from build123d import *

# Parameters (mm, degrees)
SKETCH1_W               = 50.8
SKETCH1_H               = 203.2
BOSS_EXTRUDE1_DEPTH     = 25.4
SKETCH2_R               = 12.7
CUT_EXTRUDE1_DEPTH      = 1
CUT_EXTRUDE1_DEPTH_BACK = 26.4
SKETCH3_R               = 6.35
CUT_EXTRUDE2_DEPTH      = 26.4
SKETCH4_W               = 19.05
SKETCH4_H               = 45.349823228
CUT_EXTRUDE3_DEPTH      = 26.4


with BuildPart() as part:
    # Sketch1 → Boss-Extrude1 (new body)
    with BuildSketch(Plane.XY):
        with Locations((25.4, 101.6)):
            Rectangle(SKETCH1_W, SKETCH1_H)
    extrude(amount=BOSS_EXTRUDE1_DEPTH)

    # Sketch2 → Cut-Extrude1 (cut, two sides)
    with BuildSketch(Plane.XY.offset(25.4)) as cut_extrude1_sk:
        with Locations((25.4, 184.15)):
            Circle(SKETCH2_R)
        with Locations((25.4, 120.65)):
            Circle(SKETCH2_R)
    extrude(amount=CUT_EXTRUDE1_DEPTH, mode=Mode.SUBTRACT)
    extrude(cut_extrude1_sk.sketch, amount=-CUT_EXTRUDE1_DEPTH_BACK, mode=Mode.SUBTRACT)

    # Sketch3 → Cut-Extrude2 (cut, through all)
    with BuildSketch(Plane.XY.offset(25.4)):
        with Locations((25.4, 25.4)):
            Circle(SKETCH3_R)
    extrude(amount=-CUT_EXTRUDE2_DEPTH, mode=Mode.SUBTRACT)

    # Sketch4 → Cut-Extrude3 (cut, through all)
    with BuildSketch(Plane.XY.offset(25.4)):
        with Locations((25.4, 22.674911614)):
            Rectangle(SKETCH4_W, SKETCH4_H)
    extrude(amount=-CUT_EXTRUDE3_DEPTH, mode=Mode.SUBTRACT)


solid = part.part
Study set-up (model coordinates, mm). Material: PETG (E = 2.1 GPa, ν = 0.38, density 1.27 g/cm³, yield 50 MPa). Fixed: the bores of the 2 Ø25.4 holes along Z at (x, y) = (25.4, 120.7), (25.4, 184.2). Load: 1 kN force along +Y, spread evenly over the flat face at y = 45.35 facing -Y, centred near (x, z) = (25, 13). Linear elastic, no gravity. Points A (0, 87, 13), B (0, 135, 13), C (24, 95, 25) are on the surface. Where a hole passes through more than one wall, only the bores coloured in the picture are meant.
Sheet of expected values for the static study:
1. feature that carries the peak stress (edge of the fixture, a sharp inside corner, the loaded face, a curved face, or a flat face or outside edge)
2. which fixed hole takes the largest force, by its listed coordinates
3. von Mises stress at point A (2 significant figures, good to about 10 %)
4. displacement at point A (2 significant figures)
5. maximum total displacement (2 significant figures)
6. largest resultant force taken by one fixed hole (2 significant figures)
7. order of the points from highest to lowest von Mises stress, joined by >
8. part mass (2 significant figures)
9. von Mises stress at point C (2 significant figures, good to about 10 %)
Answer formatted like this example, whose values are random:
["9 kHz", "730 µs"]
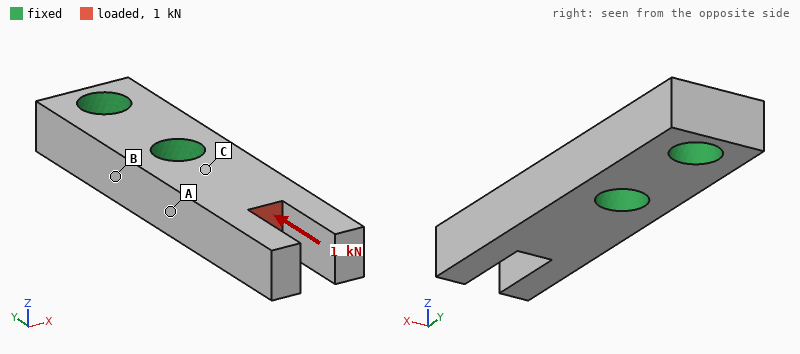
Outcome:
["a flat face or outside edge", "(25.4, 120.7)", "0.59 MPa", "12 µm", "51 µm", "960 N", "C > A > B", "270 g", "1.0 MPa"]
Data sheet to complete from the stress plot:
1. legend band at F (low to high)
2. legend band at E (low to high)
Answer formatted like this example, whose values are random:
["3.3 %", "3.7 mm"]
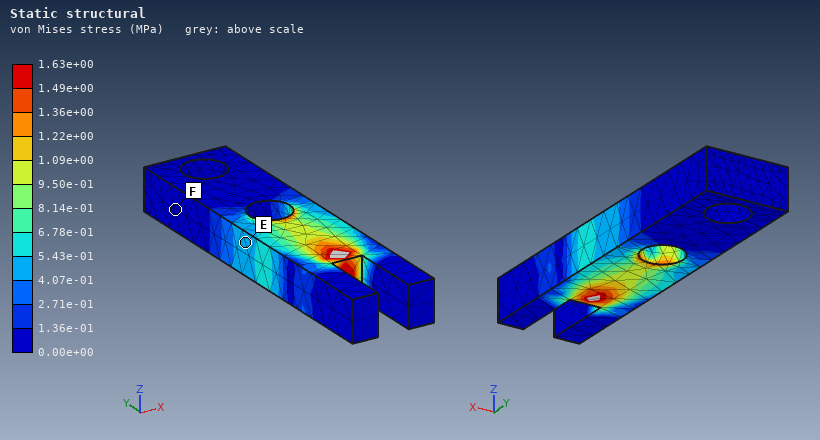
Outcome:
["0.00e+00 to 1.36e-01 MPa", "4.07e-01 to 5.43e-01 MPa"]
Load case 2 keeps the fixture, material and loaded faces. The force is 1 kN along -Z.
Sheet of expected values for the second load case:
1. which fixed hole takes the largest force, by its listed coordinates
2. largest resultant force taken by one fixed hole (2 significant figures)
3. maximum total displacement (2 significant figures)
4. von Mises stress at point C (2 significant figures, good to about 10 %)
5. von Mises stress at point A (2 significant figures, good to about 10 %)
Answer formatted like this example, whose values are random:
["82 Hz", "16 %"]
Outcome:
["(25.4, 120.7)", "1.1 kN", "1.5 mm", "10.0 MPa", "1.7 MPa"]
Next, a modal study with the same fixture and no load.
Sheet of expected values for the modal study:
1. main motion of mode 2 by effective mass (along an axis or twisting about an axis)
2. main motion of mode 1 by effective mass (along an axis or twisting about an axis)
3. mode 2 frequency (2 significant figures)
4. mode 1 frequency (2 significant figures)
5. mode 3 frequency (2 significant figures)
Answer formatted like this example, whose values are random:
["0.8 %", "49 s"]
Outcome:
["along X", "along Z", "670 Hz", "490 Hz", "1000 Hz"]
